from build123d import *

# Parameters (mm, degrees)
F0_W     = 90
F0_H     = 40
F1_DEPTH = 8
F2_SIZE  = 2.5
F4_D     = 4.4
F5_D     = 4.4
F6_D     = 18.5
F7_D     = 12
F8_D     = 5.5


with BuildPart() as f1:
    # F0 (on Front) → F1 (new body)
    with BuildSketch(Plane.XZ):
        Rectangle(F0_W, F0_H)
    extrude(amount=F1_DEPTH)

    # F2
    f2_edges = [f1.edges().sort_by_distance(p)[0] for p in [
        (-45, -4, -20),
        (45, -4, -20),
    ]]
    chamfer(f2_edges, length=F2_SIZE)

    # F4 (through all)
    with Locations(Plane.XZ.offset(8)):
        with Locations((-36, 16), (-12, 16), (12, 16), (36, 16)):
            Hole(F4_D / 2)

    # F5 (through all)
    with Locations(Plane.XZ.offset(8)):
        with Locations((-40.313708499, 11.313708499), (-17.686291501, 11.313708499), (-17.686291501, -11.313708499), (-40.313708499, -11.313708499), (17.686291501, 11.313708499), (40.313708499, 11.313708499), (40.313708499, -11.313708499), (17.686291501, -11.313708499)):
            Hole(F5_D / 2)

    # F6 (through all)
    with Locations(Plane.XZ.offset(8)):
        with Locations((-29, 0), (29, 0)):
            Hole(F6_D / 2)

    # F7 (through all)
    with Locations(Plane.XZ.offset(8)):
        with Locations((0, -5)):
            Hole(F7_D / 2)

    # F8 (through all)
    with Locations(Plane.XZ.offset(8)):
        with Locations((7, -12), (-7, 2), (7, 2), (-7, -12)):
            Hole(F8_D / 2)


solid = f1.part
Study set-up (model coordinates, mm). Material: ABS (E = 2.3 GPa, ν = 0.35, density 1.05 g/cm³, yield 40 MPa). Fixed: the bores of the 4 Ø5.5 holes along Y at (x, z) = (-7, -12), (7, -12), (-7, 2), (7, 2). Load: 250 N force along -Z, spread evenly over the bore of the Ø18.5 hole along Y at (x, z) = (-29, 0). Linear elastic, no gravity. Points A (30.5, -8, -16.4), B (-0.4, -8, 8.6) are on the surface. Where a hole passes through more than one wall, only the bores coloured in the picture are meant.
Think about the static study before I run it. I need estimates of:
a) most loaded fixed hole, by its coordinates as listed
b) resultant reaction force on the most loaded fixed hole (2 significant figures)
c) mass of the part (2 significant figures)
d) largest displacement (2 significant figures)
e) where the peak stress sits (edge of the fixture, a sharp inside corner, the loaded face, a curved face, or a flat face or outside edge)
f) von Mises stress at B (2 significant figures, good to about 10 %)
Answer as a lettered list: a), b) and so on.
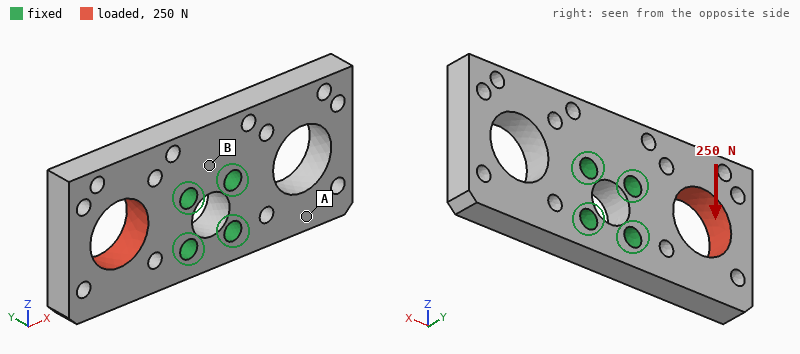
a) (-7, 2)
b) 260 N
c) 22 g
d) 0.12 mm
e) a curved face
f) 1.4 MPa
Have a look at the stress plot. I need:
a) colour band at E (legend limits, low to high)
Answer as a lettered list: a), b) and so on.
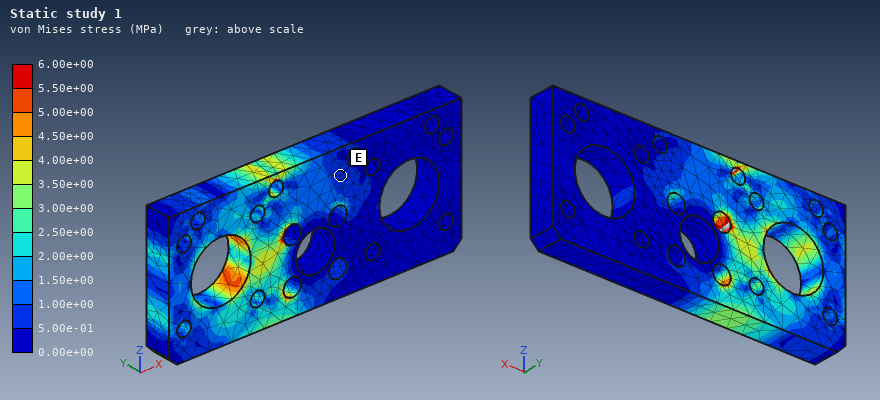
a) 5.00e-01 to 1.00e+00 MPa
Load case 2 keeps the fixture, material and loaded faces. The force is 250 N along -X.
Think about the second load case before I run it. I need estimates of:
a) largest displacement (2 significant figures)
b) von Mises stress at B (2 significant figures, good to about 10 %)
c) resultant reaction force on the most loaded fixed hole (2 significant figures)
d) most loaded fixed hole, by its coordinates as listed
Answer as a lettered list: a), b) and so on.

a) 34 µm
b) 0.74 MPa
c) 130 N
d) (-7, 2)
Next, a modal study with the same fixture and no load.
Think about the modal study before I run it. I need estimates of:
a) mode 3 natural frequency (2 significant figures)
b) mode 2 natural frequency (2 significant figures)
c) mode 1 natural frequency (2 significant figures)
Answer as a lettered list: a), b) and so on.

a) 2200 Hz
b) 1200 Hz
c) 1200 Hz
